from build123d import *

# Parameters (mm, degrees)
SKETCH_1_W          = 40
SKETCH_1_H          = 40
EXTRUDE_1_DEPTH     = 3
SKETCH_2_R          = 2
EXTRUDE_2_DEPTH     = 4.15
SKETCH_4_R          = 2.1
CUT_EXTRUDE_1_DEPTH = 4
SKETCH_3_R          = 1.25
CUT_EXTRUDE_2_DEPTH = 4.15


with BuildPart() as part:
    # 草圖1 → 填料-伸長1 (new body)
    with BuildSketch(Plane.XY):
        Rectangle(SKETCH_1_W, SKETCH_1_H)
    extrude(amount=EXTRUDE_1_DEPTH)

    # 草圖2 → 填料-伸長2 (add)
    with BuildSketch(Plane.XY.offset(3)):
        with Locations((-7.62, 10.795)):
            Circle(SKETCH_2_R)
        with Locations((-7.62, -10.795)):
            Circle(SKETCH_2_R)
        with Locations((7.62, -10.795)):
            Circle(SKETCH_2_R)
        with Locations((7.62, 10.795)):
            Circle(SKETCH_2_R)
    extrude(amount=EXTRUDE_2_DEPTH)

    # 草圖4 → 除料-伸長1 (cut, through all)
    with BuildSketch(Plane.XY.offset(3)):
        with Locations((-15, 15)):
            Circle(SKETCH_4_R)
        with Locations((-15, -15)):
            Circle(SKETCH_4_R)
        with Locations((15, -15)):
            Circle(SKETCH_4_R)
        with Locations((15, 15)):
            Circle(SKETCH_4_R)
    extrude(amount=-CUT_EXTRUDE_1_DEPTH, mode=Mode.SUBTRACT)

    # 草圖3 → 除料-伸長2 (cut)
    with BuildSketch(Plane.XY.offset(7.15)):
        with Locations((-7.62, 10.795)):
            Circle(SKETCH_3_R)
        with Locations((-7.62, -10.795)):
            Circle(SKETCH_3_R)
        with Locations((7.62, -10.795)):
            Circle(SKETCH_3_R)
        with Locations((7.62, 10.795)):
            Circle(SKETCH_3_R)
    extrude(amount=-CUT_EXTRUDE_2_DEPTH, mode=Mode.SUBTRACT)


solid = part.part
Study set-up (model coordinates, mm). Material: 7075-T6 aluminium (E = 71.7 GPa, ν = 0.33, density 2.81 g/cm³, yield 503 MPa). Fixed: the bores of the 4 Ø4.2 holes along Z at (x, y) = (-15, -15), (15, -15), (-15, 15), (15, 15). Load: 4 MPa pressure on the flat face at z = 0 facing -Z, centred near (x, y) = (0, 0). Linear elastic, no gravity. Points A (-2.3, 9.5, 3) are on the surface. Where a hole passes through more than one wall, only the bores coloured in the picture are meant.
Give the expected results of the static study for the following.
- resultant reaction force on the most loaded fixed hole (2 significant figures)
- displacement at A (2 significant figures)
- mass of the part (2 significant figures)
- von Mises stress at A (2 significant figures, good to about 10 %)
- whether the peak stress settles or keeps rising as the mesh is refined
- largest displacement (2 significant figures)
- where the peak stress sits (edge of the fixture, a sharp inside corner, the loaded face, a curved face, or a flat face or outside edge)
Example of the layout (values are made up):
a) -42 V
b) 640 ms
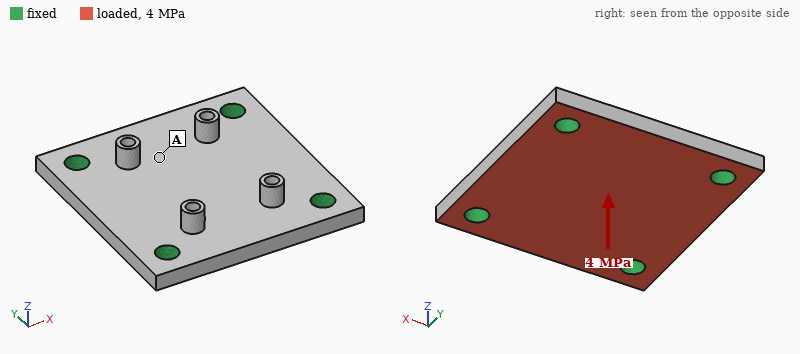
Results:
a) 1.5 kN
b) 0.076 mm
c) 13 g
d) 90 MPa
e) keeps rising
f) 0.10 mm
g) edge of the fixture
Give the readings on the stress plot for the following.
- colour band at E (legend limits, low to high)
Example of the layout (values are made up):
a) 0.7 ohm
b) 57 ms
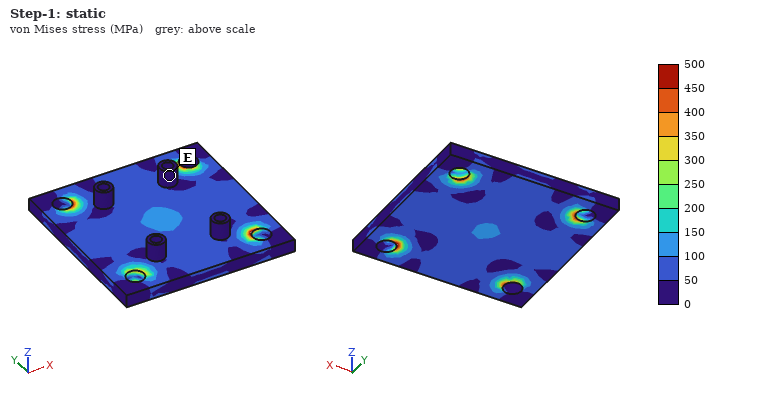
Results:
a) 0 to 50 MPa
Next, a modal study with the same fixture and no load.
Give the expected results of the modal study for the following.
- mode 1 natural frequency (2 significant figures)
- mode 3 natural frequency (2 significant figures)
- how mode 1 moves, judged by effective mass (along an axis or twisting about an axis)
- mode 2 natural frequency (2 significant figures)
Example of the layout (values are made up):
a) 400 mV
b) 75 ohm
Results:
a) 13 kHz
b) 20 kHz
c) along Z
d) 20 kHz
